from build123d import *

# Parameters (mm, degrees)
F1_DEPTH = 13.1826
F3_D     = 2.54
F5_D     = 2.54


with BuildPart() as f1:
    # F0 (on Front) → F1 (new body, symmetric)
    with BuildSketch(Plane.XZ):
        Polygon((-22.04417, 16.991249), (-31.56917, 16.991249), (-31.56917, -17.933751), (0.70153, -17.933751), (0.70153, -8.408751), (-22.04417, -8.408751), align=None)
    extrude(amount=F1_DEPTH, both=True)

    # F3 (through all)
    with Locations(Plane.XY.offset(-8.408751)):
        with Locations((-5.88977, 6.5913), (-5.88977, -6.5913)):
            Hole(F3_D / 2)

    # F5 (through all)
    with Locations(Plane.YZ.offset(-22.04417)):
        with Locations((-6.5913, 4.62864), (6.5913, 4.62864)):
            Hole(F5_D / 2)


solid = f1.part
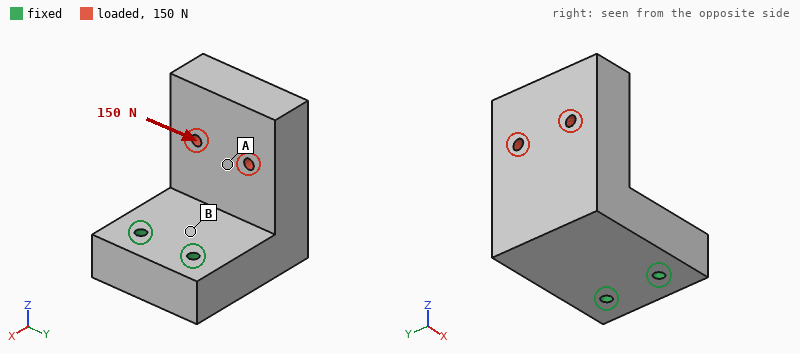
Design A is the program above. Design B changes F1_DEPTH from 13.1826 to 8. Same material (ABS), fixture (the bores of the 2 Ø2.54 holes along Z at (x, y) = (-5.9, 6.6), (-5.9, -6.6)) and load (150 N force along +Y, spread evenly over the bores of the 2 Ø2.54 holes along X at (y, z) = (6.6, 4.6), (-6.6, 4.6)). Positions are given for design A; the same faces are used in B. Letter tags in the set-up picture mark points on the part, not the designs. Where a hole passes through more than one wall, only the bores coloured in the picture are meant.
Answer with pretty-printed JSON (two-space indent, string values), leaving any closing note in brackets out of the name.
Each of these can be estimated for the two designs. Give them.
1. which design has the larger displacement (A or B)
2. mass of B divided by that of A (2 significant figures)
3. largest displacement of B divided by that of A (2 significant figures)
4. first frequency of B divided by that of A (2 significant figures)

{
  "which design has the larger displacement": "B",
  "mass of B divided by that of A": "0.60",
  "largest displacement of B divided by that of A": "2.4",
  "first frequency of B divided by that of A": "1.0"
}
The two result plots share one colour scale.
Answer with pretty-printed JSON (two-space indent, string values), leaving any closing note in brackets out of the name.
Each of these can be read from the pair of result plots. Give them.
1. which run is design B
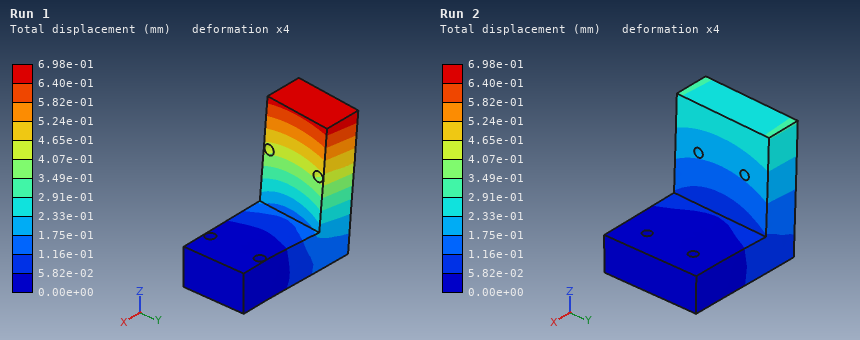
{
  "which run is design B": "Run 1"
}
